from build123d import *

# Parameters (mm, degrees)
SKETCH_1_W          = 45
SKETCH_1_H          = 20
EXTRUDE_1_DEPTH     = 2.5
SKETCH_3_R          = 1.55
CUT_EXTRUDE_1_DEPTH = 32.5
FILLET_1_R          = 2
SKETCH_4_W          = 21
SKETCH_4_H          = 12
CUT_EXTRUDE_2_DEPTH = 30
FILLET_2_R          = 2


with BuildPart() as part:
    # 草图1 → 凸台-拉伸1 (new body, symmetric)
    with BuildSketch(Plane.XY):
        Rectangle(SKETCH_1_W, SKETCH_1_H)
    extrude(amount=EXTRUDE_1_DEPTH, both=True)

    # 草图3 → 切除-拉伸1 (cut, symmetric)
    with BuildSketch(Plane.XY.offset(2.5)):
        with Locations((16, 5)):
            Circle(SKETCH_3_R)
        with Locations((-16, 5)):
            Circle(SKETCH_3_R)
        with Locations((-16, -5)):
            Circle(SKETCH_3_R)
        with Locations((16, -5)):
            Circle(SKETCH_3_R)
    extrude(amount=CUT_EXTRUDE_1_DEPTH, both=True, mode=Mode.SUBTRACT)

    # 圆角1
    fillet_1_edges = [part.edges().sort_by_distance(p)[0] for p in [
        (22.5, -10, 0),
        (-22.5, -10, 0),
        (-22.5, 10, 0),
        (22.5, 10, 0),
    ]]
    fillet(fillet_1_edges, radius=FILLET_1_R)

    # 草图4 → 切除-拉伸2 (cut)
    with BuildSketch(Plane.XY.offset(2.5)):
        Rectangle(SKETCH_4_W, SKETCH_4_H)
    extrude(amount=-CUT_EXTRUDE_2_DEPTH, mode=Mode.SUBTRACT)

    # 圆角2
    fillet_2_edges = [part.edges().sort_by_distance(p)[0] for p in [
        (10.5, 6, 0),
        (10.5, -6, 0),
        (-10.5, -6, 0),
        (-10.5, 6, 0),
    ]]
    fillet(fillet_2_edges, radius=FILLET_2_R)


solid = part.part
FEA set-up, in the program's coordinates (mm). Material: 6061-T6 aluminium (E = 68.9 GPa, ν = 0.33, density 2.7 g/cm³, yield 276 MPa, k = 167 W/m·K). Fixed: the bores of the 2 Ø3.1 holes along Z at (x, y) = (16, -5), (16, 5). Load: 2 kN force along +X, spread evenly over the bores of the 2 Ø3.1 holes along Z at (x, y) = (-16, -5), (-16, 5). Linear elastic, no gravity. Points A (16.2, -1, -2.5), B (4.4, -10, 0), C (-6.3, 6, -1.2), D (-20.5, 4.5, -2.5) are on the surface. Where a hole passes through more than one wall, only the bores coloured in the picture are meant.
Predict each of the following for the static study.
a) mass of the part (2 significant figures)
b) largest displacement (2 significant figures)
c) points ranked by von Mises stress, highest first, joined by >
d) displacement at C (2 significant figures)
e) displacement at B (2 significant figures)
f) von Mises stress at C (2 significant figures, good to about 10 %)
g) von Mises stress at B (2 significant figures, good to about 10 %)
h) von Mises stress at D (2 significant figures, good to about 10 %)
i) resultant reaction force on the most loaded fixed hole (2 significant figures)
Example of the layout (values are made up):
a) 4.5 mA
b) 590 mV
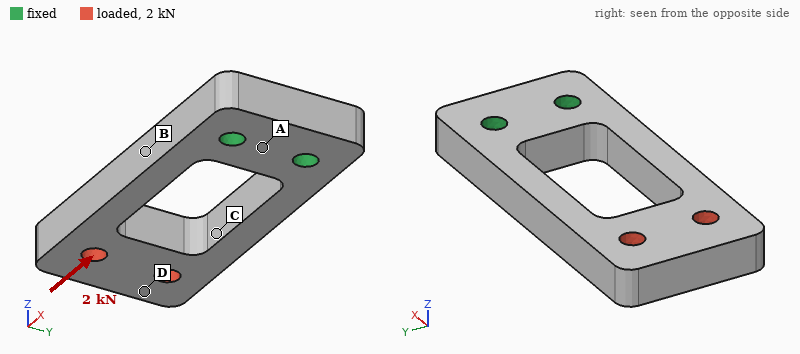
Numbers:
a) 8.3 g
b) 27 µm
c) C > B > D > A
d) 19 µm
e) 13 µm
f) 68 MPa
g) 37 MPa
h) 21 MPa
i) 1.0 kN
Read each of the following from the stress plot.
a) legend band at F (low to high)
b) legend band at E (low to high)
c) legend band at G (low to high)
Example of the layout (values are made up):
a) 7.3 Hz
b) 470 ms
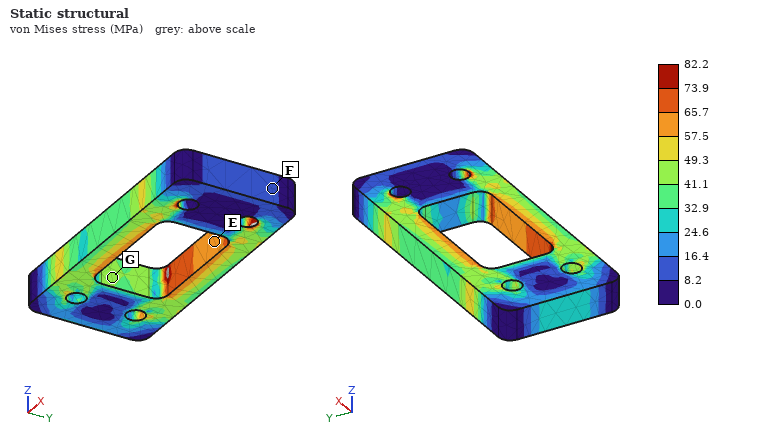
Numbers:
a) 8.2 to 16.4 MPa
b) 57.5 to 65.7 MPa
c) 41.1 to 49.3 MPa
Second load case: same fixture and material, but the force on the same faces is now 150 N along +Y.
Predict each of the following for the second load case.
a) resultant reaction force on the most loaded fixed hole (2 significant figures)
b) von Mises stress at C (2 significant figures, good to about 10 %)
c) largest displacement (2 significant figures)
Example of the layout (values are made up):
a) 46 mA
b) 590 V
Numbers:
a) 340 N
b) 42 MPa
c) 64 µm
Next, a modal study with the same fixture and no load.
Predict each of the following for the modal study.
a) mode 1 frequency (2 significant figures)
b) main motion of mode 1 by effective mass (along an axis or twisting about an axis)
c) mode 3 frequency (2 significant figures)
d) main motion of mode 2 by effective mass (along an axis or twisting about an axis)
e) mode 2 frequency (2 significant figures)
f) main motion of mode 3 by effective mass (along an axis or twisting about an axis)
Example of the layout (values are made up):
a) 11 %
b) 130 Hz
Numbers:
a) 2100 Hz
b) along Z
c) 6600 Hz
d) along Y
e) 4100 Hz
f) twisting about X
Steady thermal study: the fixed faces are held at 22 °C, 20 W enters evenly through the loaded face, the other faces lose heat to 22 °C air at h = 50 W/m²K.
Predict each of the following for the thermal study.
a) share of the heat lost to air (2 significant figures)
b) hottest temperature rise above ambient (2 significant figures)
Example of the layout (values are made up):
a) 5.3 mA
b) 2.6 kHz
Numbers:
a) 19 %
b) 71 K
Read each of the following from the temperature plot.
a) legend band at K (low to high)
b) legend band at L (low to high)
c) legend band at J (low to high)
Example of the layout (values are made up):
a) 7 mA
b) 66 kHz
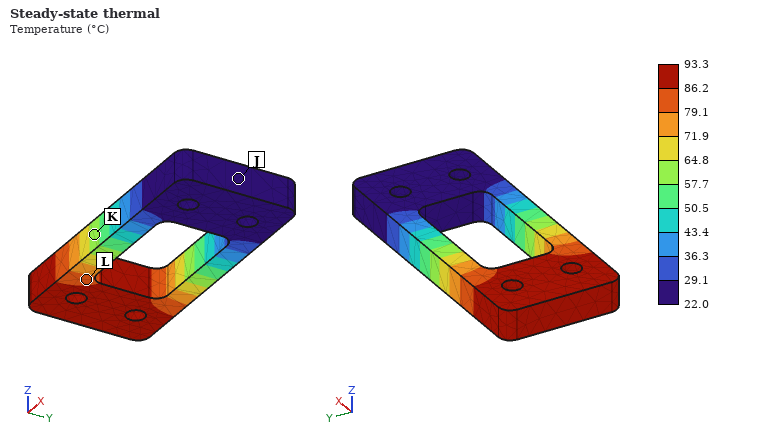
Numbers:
a) 57.7 to 64.8 °C
b) 79.1 to 86.2 °C
c) 22.0 to 29.1 °C
